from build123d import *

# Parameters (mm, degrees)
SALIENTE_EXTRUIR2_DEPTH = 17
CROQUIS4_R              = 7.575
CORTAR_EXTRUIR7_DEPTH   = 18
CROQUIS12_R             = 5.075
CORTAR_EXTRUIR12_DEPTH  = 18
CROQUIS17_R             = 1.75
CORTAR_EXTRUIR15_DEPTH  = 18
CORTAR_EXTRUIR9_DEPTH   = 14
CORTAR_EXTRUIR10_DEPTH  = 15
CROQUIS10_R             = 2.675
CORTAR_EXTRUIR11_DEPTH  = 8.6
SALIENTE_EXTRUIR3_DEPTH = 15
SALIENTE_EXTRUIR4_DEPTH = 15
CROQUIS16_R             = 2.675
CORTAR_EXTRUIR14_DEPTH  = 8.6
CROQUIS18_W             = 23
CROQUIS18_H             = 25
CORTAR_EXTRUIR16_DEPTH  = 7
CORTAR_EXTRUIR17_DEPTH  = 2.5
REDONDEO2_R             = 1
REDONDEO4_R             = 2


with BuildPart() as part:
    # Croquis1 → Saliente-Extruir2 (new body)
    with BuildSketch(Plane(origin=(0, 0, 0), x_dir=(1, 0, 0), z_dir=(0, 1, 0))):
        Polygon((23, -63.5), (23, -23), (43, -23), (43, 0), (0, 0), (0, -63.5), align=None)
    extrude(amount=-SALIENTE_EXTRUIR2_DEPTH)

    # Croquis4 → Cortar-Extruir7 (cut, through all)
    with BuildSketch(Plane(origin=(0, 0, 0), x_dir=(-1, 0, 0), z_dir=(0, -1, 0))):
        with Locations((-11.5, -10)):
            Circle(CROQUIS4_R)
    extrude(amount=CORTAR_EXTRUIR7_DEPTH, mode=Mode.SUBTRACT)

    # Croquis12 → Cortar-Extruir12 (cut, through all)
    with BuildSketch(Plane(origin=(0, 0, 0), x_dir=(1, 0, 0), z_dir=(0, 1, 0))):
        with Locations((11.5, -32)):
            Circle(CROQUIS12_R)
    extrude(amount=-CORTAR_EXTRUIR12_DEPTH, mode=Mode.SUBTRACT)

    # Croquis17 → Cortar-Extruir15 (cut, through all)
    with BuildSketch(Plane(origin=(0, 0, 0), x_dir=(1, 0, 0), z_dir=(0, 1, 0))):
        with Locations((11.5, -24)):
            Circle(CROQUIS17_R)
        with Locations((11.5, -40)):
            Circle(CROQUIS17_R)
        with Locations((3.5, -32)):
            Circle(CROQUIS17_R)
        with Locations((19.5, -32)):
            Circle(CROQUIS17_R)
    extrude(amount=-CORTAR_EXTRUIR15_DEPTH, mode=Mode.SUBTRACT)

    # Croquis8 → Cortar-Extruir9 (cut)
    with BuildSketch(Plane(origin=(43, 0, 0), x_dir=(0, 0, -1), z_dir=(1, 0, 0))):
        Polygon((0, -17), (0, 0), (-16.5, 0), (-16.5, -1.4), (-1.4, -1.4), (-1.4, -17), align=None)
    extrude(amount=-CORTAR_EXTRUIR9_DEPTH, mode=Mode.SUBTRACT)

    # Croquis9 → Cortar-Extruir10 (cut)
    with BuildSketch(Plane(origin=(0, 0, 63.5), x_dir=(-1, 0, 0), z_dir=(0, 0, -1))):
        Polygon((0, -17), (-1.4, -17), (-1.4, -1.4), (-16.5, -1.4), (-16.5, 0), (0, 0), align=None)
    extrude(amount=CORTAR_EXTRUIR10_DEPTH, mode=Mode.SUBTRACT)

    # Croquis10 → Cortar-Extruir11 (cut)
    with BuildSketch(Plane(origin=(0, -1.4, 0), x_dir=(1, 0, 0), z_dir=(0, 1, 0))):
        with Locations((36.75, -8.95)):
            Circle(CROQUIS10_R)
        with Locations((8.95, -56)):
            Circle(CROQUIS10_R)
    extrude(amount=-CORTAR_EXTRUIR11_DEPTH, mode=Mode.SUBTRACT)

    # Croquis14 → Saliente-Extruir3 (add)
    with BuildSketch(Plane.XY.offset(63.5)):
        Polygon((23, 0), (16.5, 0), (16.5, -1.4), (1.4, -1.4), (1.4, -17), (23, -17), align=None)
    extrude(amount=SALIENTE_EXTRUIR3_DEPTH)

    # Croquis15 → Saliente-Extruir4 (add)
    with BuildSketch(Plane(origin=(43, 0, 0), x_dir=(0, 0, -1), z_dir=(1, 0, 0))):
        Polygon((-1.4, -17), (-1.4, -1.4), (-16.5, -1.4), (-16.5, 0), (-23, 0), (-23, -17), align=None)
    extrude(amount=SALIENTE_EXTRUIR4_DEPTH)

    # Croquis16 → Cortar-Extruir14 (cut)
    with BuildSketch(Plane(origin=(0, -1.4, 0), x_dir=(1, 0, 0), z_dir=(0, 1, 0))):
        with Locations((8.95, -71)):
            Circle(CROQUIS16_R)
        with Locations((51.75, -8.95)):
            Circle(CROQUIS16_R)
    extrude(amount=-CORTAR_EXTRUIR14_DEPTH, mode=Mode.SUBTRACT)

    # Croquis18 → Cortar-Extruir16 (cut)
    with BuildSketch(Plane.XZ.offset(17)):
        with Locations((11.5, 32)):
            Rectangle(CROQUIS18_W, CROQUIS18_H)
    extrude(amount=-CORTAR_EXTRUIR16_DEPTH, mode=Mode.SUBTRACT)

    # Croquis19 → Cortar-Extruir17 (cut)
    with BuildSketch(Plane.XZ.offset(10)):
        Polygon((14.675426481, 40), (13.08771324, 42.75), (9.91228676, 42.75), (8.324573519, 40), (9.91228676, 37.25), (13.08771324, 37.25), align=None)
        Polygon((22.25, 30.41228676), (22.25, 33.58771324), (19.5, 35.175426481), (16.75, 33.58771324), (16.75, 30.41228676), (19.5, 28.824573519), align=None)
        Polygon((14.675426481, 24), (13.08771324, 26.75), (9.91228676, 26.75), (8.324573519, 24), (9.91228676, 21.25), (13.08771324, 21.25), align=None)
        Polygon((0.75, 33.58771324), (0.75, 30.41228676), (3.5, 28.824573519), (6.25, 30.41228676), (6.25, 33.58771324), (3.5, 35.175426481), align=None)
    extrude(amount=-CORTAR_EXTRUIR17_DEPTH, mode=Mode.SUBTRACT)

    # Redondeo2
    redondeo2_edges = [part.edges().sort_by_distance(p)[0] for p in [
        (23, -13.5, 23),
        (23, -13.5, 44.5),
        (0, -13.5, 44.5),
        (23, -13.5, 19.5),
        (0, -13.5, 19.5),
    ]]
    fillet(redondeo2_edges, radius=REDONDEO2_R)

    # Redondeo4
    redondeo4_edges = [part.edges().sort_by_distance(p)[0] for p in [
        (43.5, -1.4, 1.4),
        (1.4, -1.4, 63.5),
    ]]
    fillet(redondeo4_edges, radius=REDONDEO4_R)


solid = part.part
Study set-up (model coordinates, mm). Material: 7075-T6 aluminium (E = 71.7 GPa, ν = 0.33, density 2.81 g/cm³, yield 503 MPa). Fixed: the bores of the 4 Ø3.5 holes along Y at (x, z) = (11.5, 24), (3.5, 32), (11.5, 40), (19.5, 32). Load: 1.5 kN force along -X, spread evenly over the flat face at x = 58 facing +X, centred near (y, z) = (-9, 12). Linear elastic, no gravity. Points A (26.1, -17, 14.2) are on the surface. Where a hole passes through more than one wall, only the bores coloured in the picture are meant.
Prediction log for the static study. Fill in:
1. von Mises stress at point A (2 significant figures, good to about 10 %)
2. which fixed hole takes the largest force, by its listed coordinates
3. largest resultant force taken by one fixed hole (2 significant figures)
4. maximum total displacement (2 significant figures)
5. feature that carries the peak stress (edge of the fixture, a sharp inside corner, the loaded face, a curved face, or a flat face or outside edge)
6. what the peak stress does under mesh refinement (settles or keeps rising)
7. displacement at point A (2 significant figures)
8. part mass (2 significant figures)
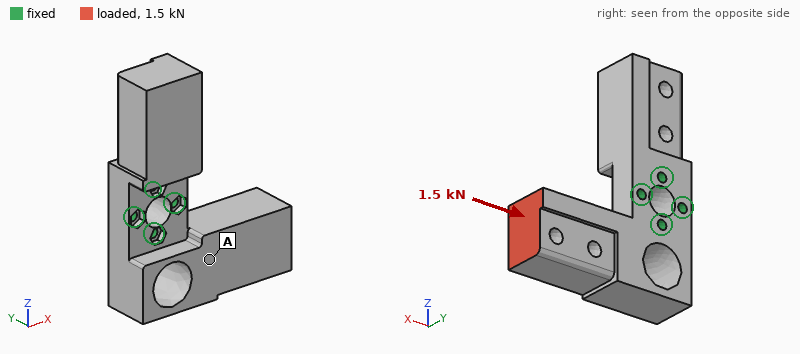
8.2 MPa
(11.5, 24)
1.7 kN
49 µm
edge of the fixture
keeps rising
18 µm
91 g
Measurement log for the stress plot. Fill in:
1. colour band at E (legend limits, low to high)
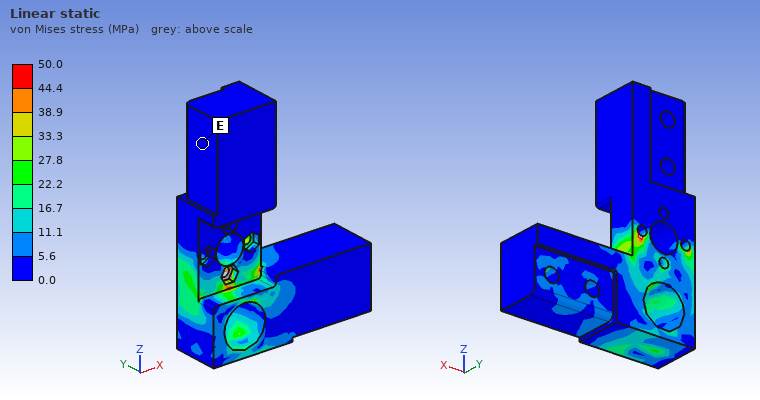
0.0 to 5.6 MPa
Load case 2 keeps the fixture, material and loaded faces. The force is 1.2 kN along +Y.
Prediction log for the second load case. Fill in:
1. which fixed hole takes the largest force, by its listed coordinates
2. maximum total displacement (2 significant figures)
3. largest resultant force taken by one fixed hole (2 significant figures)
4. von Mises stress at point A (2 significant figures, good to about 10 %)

(19.5, 32)
0.37 mm
1.6 kN
55 MPa
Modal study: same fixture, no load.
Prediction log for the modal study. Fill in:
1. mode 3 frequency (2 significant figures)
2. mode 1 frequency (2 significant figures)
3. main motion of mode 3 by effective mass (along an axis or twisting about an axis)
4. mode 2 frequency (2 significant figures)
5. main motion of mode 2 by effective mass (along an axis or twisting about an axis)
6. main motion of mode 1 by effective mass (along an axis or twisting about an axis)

3800 Hz
2500 Hz
along Y
3500 Hz
along Z
along Y
